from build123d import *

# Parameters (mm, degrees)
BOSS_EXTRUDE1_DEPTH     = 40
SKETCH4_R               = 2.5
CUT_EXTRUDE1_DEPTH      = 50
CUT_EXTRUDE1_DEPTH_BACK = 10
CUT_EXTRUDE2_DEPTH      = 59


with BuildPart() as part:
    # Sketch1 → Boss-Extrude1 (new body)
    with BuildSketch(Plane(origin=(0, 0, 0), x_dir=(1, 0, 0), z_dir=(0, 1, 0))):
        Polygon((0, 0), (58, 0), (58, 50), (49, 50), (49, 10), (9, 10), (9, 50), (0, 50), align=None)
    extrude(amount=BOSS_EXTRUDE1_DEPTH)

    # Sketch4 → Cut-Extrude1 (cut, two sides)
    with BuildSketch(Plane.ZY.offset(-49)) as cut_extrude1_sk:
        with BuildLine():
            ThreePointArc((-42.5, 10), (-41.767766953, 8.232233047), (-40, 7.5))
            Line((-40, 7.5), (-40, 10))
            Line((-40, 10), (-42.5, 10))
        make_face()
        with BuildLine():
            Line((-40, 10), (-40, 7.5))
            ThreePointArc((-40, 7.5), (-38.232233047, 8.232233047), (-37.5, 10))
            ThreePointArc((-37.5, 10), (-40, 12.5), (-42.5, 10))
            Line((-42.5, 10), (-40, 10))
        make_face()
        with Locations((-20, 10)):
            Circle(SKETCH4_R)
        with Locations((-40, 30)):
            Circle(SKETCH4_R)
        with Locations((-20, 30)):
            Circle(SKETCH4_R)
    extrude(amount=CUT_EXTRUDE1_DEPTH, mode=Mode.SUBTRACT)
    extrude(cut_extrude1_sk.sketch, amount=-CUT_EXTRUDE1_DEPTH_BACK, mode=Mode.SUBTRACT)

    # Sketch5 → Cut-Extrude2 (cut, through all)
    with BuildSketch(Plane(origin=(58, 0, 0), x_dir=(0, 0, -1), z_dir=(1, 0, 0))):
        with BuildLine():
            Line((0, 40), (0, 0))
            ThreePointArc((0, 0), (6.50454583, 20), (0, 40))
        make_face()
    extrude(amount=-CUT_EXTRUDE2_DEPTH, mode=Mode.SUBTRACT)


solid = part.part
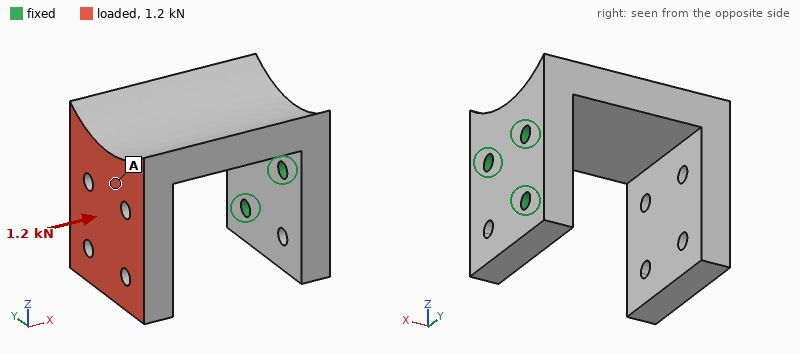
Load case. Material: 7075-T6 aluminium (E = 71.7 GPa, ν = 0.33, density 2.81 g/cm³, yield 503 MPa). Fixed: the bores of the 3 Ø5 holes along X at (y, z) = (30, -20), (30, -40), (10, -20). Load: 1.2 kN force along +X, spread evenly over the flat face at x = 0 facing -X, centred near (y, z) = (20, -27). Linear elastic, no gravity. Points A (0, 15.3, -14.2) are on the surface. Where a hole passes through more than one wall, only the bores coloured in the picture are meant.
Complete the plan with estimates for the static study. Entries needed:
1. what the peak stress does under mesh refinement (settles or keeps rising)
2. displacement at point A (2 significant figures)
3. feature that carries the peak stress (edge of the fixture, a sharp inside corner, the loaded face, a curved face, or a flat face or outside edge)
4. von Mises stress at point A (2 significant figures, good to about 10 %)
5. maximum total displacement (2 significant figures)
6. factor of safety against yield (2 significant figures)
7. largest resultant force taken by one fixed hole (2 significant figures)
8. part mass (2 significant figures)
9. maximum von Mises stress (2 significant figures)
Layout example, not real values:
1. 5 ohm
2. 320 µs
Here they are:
1. settles
2. 0.55 mm
3. a curved face
4. 28 MPa
5. 0.97 mm
6. 3.2
7. 620 N
8. 110 g
9. 160 MPa
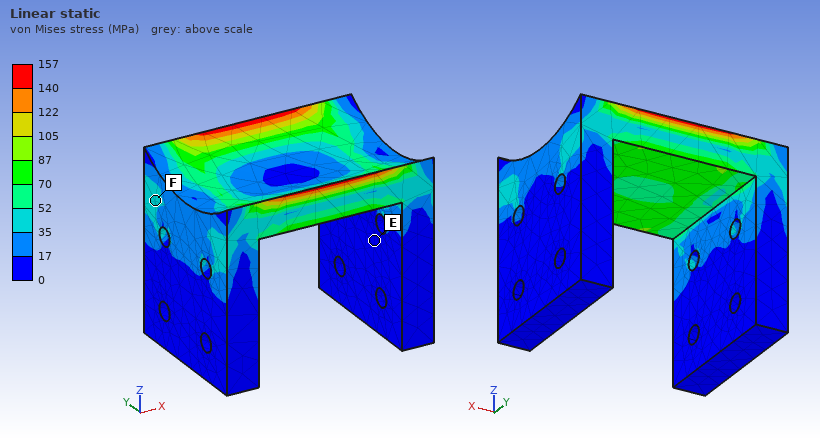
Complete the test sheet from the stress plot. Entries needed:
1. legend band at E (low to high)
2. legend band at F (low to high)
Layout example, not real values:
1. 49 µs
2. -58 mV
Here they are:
1. 0 to 17 MPa
2. 35 to 52 MPa
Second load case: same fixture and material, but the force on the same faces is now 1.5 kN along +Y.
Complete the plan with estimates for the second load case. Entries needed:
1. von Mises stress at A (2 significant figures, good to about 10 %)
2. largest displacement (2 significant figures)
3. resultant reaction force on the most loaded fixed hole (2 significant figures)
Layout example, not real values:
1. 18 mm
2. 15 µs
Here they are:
1. 25 MPa
2. 0.91 mm
3. 3.2 kN
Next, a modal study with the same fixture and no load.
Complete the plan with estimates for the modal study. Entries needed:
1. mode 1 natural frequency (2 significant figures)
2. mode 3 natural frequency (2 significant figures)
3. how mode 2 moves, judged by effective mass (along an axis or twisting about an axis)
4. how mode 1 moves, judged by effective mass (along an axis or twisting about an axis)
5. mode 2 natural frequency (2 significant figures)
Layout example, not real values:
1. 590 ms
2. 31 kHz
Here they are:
1. 710 Hz
2. 2200 Hz
3. along Y
4. along Z
5. 1100 Hz
